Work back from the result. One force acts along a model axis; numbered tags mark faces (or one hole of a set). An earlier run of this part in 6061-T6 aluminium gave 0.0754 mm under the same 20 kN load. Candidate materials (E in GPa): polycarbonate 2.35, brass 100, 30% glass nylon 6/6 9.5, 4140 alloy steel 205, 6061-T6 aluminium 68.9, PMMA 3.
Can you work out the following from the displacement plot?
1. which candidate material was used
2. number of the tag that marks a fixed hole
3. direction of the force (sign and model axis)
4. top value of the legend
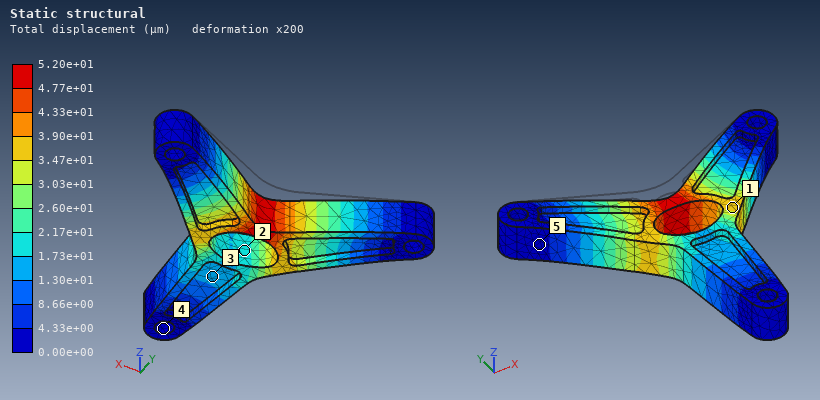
brass
4
-Y
5.20e+01 µm
